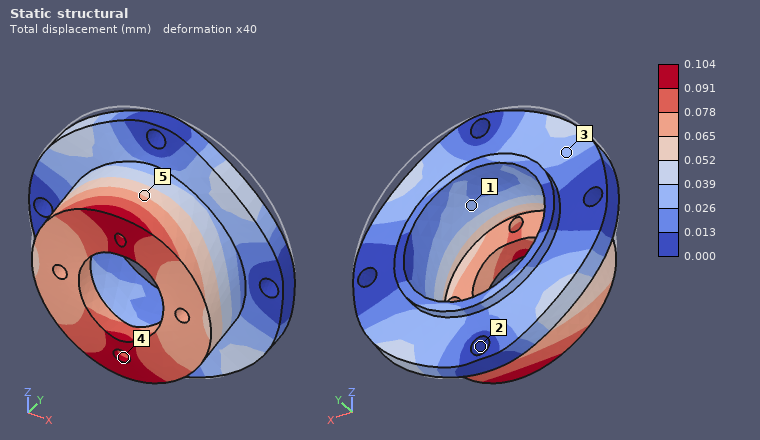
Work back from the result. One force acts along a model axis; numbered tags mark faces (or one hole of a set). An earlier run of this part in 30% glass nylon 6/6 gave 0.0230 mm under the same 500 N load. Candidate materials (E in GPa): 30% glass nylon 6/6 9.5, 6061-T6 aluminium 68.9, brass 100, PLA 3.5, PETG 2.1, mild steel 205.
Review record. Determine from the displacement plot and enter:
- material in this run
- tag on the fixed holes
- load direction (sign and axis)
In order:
PETG
2
-Z
